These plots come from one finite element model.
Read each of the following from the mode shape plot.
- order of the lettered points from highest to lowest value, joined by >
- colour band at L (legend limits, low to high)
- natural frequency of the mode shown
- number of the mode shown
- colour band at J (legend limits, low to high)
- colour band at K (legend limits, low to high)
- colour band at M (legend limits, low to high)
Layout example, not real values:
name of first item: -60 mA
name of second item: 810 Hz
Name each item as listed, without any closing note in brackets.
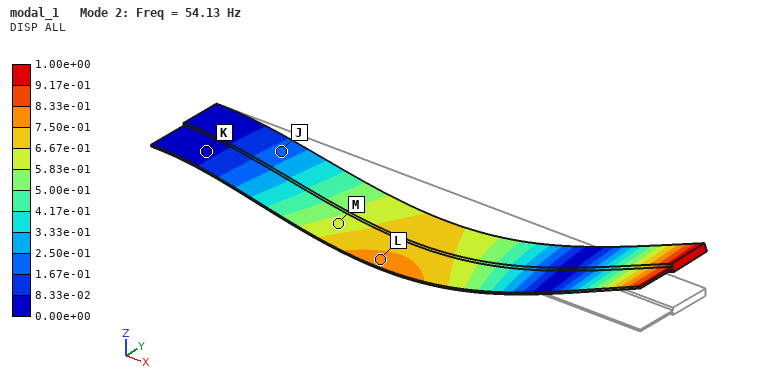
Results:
order of the lettered points from highest to lowest value, joined by >: L > M > J > K
colour band at L: 7.50e-01 to 8.33e-01
natural frequency of the mode shown: 54.13 Hz
number of the mode shown: 2
colour band at J: 1.67e-01 to 2.50e-01
colour band at K: 0.00e+00 to 8.33e-02
colour band at M: 5.83e-01 to 6.67e-01
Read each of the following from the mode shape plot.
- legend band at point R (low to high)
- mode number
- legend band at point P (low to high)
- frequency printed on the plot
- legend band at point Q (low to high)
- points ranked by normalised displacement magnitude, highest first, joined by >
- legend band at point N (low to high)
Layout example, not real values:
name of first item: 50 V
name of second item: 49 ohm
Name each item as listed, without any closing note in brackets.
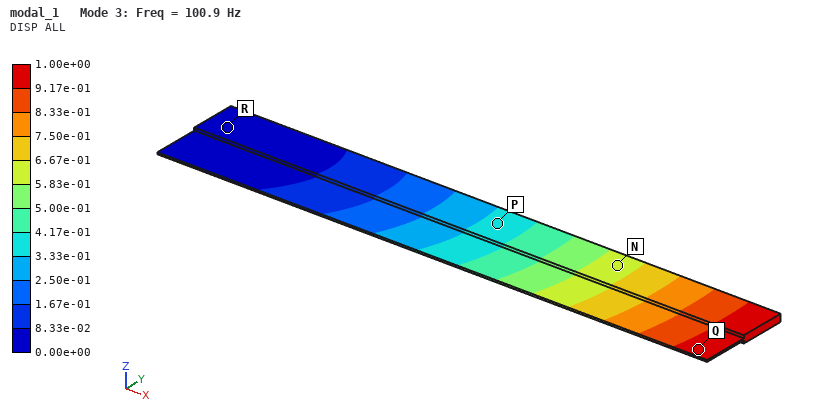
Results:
legend band at point R: 0.00e+00 to 8.33e-02
mode number: 3
legend band at point P: 3.33e-01 to 4.17e-01
frequency printed on the plot: 100.9 Hz
legend band at point Q: 9.17e-01 to 1.00e+00
points ranked by normalised displacement magnitude, highest first, joined by >: Q > N > P > R
legend band at point N: 5.83e-01 to 6.67e-01
